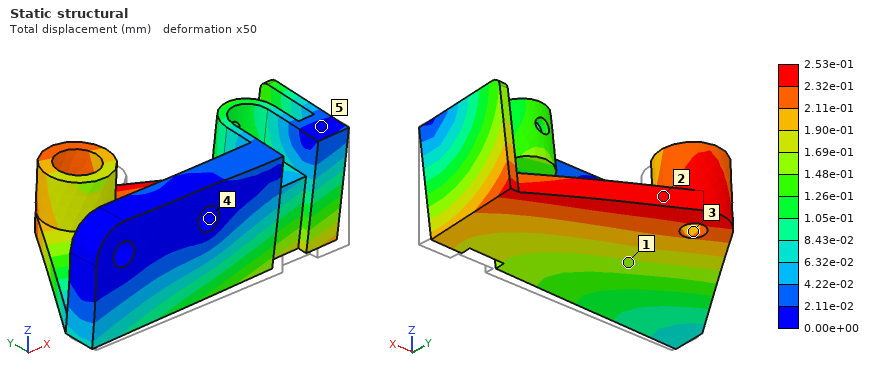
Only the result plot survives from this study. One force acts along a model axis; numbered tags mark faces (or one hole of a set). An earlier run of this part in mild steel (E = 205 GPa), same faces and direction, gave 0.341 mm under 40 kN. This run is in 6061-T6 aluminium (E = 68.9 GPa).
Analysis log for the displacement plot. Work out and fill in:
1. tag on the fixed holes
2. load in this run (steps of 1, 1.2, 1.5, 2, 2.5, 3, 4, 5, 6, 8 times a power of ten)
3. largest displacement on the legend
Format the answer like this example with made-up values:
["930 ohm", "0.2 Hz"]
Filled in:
["4", "10 kN", "2.53e-01 mm"]
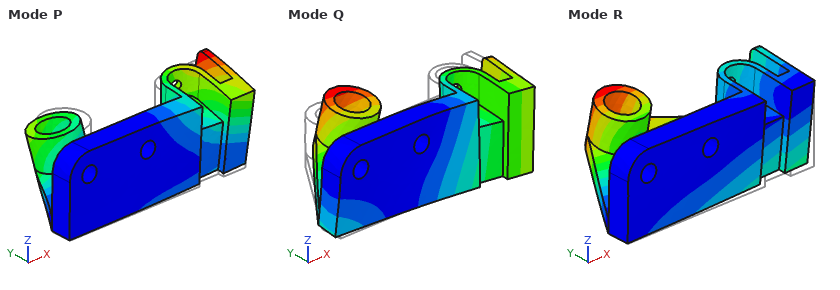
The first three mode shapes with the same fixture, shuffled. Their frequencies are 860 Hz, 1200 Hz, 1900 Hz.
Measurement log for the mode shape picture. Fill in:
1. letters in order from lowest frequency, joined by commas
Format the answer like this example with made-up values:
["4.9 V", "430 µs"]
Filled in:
["R, Q, P"]
